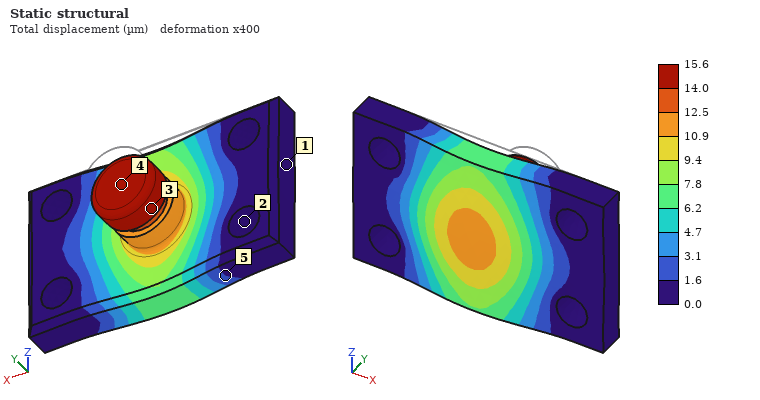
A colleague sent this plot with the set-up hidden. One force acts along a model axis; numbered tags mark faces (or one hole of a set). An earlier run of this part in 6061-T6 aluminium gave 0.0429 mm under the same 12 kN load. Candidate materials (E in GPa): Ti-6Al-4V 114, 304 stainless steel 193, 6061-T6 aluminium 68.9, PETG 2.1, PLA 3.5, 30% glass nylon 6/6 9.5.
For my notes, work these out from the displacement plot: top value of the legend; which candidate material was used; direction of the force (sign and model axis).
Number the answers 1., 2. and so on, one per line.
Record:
1. 15.6 µm
2. 304 stainless steel
3. -Y
